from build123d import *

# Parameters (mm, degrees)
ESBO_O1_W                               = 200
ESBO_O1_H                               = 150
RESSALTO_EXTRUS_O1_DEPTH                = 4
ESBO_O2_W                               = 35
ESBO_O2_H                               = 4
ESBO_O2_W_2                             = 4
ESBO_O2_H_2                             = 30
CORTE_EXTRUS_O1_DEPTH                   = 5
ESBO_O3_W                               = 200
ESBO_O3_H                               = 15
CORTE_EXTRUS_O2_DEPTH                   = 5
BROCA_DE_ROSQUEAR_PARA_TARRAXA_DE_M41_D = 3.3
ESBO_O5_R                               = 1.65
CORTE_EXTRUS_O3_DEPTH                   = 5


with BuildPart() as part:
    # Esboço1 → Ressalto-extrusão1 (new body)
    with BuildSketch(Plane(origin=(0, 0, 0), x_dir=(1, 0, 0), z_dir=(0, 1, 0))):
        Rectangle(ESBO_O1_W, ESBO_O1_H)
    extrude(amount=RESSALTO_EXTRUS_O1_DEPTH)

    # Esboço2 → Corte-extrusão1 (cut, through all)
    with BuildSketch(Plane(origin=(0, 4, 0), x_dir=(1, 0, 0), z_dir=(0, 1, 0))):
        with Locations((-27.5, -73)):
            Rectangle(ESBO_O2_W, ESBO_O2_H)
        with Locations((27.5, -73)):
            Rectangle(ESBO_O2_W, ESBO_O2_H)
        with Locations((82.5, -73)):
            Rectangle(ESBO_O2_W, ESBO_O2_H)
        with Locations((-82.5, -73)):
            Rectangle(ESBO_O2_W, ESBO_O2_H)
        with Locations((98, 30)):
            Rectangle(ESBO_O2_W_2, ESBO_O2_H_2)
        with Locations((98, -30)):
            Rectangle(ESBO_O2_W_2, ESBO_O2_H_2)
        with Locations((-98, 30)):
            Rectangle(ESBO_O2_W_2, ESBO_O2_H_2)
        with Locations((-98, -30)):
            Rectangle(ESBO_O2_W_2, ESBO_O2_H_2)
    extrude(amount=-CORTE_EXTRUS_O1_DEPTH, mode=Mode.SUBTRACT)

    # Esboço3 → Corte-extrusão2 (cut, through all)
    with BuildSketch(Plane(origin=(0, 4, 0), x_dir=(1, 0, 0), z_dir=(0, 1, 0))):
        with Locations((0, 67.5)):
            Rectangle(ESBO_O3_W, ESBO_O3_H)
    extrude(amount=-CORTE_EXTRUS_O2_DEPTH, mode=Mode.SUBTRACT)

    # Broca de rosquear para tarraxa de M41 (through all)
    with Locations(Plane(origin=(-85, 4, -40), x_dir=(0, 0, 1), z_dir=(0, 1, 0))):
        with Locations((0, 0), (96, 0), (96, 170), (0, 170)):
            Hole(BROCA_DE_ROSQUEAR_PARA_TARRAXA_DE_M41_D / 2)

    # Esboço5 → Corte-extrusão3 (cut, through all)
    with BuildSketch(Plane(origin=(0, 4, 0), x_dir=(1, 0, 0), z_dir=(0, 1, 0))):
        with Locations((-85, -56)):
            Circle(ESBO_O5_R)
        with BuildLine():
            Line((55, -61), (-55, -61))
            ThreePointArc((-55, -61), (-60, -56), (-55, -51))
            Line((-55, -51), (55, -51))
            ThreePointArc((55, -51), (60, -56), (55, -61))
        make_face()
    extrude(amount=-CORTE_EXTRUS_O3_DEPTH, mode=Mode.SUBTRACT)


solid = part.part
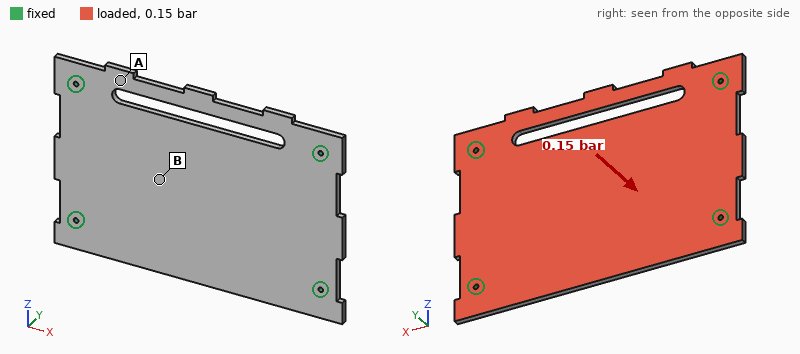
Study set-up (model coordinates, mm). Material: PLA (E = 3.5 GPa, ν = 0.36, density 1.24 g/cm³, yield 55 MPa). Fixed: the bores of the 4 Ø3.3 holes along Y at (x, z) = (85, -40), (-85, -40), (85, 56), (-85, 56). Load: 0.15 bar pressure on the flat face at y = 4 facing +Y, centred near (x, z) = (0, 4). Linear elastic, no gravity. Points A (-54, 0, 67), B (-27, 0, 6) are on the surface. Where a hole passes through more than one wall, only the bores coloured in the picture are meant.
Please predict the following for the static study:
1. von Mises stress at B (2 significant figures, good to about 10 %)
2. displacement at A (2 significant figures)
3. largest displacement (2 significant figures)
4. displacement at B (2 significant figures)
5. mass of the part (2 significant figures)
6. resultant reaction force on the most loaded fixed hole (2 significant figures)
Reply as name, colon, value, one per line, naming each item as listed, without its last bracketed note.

von Mises stress at B: 5.6 MPa
displacement at A: 0.81 mm
largest displacement: 2.7 mm
displacement at B: 2.2 mm
mass of the part: 120 g
resultant reaction force on the most loaded fixed hole: 99 N
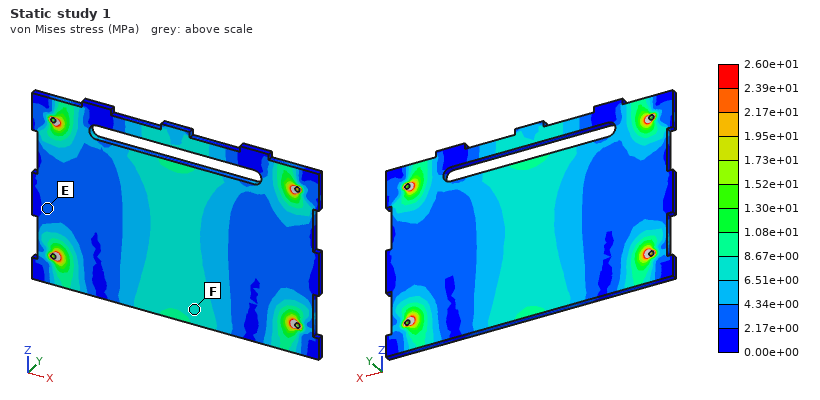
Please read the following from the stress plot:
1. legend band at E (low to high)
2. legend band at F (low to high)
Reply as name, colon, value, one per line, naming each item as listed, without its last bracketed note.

legend band at E: 2.17e+00 to 4.34e+00 MPa
legend band at F: 6.51e+00 to 8.67e+00 MPa
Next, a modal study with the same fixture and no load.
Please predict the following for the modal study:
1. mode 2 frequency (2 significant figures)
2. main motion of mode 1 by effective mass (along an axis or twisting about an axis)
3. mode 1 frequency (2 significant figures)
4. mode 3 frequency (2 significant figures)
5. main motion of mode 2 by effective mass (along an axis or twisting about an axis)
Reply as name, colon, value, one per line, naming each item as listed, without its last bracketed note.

mode 2 frequency: 290 Hz
main motion of mode 1 by effective mass: along Y
mode 1 frequency: 200 Hz
mode 3 frequency: 360 Hz
main motion of mode 2 by effective mass: twisting about X
